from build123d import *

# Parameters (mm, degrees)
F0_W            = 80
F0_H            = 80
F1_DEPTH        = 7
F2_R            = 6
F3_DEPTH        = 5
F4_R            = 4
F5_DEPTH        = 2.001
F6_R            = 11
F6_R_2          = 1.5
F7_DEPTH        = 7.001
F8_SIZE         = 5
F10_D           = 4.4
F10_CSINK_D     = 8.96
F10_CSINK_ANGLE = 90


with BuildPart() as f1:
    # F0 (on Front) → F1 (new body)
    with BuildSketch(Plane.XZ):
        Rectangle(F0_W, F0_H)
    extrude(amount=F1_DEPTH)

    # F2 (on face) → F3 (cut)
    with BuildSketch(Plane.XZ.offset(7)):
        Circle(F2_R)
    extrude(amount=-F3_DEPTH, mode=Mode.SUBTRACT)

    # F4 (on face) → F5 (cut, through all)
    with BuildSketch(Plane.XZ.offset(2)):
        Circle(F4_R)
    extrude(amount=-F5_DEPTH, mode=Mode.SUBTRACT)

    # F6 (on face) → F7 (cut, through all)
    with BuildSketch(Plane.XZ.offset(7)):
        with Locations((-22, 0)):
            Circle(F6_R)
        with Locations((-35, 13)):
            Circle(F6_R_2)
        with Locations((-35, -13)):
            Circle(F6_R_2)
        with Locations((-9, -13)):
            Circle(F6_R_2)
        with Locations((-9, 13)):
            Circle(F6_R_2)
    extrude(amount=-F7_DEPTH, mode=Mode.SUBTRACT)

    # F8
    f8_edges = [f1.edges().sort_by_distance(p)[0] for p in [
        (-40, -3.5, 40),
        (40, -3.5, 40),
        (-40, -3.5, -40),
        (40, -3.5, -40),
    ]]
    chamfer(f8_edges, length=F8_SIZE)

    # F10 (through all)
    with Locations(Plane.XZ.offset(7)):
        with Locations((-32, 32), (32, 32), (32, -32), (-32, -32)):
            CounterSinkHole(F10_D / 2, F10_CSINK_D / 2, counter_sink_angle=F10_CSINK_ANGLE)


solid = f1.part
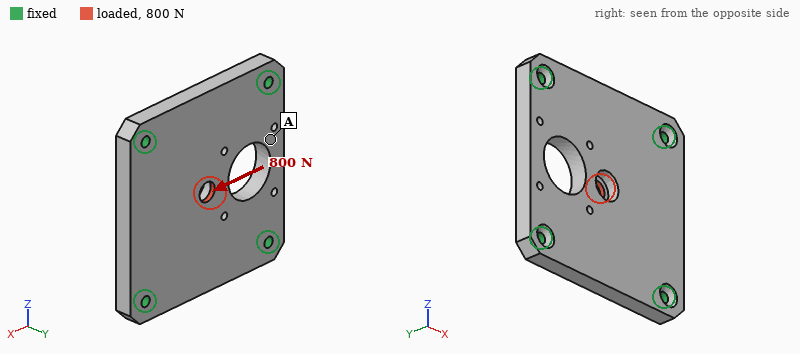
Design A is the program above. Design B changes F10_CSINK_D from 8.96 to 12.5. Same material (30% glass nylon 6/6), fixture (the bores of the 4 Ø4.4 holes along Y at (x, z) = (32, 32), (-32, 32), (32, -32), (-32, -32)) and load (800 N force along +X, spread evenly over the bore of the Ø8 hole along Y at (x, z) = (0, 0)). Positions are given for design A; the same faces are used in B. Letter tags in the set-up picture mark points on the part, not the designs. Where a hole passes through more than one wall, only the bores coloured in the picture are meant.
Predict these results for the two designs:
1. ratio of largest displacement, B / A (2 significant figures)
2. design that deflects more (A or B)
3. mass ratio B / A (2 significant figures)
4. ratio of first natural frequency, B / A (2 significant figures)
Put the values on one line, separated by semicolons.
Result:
1.1; B; 0.99; 0.90
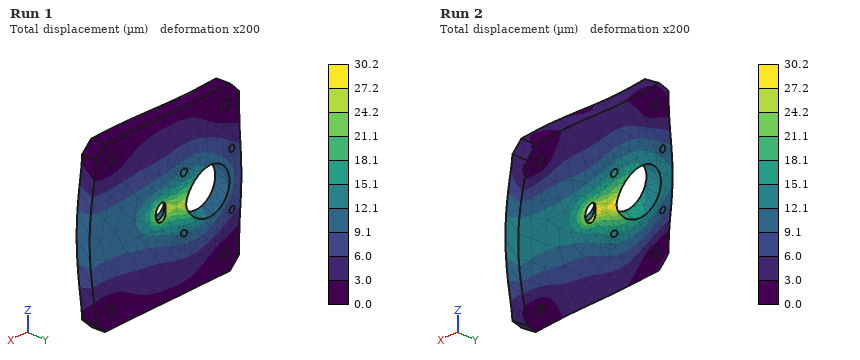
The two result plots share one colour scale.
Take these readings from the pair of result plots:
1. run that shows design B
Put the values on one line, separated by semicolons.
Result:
Run 2
